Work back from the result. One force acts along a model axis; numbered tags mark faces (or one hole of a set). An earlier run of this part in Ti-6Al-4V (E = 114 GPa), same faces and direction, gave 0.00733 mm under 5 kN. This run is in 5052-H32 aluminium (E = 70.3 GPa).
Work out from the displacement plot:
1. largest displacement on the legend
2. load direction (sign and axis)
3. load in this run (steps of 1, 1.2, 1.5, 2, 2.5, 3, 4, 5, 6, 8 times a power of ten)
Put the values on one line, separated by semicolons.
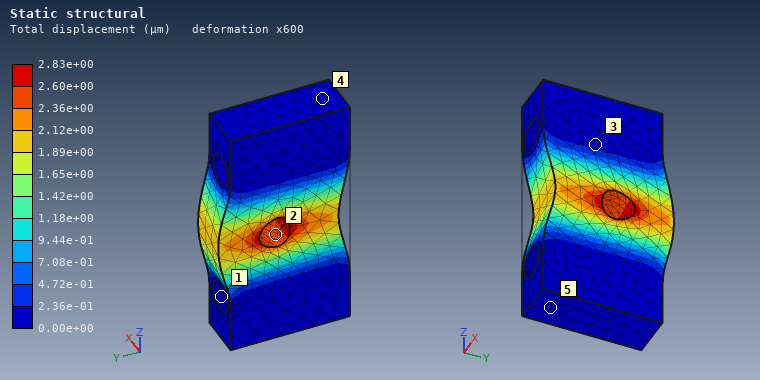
2.83e+00 µm; +Y; 1.2 kN
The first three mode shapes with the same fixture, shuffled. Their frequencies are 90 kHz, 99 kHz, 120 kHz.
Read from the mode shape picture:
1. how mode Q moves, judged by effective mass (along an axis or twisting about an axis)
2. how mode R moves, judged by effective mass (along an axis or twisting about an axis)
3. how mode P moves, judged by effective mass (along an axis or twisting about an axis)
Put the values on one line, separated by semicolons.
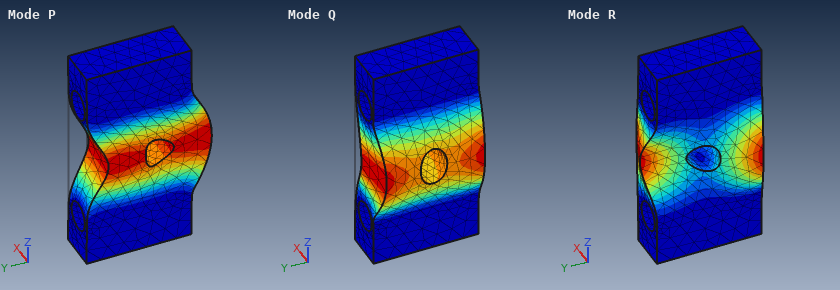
along X; twisting about Z; along Y
